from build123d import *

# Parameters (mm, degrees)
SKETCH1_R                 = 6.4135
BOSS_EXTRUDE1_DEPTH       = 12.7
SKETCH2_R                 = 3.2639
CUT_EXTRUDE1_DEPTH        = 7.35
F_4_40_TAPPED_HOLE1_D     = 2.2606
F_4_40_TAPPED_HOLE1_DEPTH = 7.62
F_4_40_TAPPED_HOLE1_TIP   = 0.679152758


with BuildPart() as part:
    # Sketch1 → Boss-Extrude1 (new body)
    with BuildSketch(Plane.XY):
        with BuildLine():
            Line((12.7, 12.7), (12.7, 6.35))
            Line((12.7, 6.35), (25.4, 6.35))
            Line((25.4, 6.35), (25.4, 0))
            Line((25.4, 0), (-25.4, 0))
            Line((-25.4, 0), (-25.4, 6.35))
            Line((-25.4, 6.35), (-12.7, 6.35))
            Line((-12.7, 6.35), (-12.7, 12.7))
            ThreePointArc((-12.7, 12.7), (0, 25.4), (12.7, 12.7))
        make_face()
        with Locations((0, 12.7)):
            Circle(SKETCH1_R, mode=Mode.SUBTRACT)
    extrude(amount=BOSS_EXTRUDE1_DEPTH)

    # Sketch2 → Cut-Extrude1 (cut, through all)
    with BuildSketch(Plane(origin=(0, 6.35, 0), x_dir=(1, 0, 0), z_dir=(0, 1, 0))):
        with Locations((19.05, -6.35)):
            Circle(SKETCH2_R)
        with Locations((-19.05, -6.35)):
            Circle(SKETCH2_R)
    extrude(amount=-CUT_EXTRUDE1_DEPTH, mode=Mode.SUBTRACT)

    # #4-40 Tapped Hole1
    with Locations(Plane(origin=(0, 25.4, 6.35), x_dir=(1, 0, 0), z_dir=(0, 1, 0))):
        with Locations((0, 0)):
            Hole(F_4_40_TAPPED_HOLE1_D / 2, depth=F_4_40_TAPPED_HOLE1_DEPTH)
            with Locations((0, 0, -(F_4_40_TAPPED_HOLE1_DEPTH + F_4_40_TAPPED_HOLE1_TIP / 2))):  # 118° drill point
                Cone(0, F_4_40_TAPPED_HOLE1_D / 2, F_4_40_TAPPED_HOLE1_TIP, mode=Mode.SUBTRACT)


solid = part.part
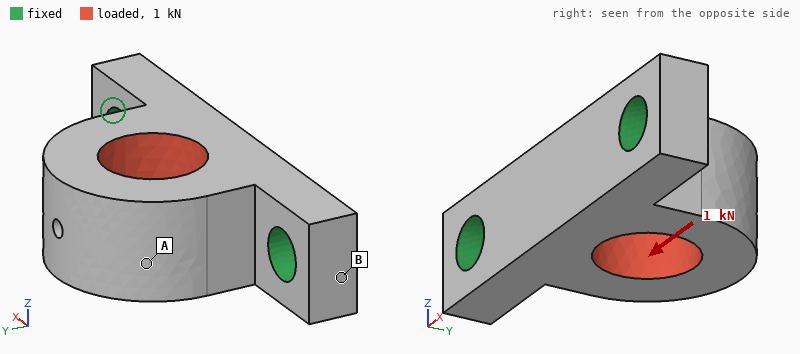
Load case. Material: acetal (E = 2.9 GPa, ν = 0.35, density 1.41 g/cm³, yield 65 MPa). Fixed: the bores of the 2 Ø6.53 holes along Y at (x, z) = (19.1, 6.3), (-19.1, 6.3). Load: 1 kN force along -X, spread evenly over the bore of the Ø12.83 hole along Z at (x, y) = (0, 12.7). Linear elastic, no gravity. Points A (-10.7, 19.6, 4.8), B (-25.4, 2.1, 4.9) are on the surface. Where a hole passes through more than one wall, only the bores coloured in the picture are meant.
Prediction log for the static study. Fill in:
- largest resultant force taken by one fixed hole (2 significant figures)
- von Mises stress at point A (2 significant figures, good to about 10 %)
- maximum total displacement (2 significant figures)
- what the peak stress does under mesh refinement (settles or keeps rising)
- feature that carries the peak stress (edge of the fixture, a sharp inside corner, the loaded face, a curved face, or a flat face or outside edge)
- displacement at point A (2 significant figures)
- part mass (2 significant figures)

590 N
5.4 MPa
0.15 mm
keeps rising
edge of the fixture
0.14 mm
10 g
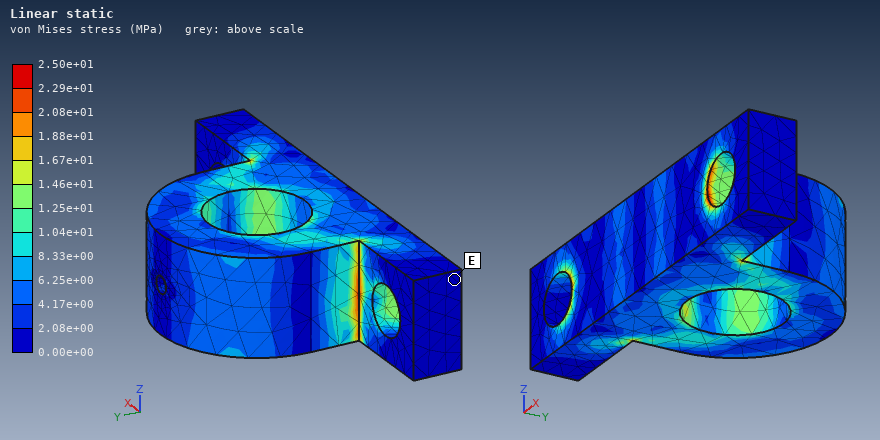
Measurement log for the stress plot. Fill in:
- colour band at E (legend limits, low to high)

0.00e+00 to 2.08e+00 MPa
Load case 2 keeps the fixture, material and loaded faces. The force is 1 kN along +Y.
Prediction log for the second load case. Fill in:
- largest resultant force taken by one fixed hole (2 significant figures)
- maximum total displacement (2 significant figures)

520 N
0.12 mm
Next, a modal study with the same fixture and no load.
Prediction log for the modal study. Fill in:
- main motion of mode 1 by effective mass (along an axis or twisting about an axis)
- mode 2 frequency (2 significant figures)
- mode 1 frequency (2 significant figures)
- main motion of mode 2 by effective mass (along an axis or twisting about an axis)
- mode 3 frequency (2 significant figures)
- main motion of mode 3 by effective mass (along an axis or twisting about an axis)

along Z
5400 Hz
2500 Hz
along X
6100 Hz
along Y
